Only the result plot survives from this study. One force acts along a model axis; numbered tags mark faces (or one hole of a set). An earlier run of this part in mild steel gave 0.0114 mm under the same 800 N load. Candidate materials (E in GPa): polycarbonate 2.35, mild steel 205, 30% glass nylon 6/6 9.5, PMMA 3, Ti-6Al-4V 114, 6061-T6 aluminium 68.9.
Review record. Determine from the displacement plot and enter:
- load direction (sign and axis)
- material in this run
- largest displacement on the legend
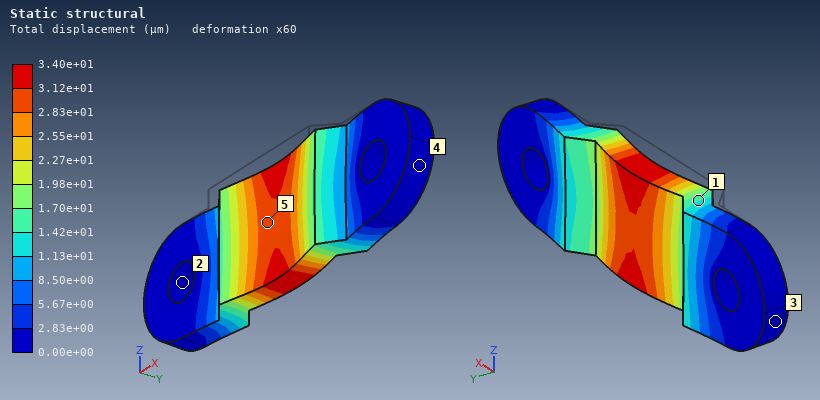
+Y
6061-T6 aluminium
3.40e+01 µm
